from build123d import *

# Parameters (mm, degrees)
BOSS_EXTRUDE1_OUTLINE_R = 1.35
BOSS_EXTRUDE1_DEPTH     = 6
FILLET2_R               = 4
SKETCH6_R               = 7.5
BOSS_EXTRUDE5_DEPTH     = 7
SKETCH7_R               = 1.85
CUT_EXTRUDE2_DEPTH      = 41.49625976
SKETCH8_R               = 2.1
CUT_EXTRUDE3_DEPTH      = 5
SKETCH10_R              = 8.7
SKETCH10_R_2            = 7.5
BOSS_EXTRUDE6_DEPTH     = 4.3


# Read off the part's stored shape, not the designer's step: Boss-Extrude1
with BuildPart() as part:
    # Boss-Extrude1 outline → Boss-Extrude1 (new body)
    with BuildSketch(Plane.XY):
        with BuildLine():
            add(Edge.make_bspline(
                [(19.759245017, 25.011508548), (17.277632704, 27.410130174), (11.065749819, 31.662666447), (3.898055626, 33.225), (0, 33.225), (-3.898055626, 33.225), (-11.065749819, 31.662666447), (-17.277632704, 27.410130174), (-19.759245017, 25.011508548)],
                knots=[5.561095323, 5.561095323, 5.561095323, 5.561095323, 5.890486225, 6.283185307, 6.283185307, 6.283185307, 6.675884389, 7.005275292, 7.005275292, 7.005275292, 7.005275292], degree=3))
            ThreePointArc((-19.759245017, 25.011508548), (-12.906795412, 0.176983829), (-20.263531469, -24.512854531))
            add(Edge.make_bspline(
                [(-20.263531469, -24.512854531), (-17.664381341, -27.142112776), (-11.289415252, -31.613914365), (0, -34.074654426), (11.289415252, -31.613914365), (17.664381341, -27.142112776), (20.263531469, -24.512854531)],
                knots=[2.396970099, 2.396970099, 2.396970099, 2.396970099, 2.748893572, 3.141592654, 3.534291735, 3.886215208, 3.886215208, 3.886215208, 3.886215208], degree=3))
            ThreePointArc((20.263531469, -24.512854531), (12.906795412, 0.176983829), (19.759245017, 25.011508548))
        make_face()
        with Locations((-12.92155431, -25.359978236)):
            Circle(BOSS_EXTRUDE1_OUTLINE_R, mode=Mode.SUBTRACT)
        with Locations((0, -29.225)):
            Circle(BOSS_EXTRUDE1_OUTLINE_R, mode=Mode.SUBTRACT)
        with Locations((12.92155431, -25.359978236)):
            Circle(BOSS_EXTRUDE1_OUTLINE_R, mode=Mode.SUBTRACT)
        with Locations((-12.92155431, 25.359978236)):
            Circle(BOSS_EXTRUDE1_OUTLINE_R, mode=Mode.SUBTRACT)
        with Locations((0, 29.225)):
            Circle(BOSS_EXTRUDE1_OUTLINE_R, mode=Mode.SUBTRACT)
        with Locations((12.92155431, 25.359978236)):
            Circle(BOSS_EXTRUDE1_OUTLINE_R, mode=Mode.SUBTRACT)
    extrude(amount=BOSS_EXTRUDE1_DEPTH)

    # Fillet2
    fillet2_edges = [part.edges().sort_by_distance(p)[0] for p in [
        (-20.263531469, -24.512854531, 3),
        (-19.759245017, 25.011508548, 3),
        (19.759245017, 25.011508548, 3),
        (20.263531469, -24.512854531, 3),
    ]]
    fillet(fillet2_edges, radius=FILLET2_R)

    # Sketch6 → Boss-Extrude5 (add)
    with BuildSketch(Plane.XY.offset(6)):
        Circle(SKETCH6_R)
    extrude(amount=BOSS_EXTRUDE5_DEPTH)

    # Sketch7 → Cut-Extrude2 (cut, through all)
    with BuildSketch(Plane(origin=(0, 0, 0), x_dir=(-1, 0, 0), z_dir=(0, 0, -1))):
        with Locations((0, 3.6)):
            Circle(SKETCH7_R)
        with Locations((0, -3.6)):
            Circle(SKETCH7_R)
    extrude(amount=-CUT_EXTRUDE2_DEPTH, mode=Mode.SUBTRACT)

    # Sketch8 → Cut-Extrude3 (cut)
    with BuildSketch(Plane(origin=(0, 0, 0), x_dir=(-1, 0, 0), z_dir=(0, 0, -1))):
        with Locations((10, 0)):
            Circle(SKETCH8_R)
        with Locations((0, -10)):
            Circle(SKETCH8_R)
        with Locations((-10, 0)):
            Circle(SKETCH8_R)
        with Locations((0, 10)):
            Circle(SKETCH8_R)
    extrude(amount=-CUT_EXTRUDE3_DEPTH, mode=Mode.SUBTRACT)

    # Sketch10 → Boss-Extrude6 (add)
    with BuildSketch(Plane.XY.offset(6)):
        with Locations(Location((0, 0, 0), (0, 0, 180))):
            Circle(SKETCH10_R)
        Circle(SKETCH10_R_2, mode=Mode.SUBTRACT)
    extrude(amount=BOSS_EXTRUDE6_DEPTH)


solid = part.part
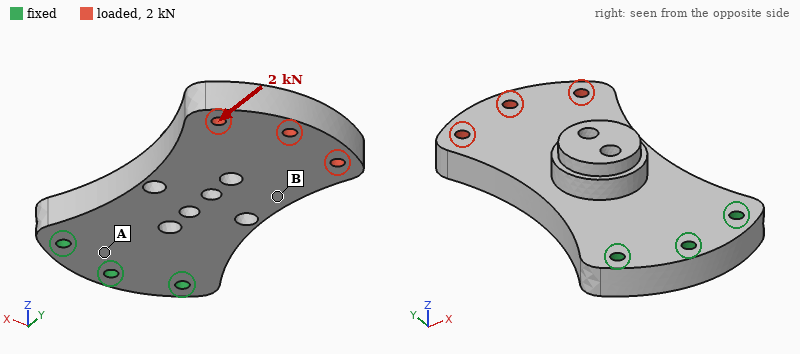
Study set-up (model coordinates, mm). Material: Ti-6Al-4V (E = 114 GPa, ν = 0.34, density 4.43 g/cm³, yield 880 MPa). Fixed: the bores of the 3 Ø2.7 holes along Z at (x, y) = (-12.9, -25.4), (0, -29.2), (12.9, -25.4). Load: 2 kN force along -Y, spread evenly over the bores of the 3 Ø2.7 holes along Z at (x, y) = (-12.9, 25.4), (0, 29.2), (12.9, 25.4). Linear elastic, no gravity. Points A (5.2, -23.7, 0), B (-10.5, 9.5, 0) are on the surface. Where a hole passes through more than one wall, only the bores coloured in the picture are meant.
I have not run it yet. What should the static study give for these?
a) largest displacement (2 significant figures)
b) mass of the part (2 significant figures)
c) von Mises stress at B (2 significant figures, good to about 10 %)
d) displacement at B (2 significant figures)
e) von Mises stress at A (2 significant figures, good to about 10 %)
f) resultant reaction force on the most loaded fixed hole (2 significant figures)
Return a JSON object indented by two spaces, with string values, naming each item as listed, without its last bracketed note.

{
  "largest displacement": "12 µm",
  "mass of the part": "55 g",
  "von Mises stress at B": "13 MPa",
  "displacement at B": "5.9 µm",
  "von Mises stress at A": "5.7 MPa",
  "resultant reaction force on the most loaded fixed hole": "720 N"
}
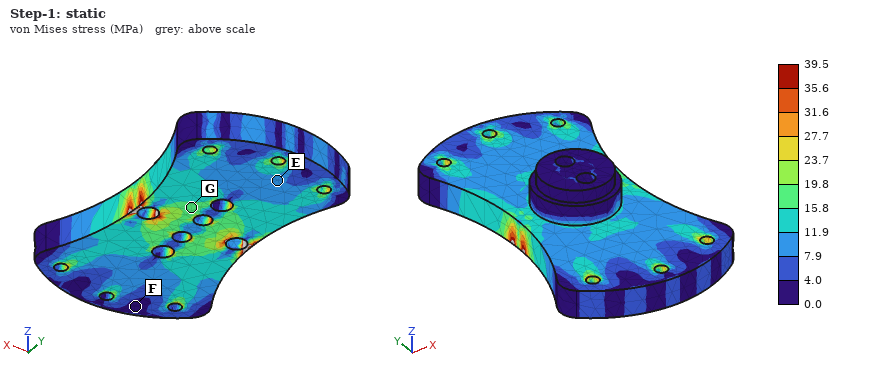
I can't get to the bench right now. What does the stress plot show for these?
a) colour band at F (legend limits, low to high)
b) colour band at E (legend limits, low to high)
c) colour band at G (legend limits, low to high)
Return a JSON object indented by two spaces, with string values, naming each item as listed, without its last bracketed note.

{
  "colour band at F": "0.0 to 4.0 MPa",
  "colour band at E": "7.9 to 11.9 MPa",
  "colour band at G": "15.8 to 19.8 MPa"
}
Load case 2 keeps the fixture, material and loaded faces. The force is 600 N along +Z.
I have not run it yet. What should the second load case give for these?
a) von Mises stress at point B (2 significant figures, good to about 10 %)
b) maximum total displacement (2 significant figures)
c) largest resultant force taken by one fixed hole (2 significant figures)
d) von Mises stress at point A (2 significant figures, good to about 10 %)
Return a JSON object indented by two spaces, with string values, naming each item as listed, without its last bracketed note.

{
  "von Mises stress at point B": "57 MPa",
  "maximum total displacement": "0.54 mm",
  "largest resultant force taken by one fixed hole": "470 N",
  "von Mises stress at point A": "94 MPa"
}
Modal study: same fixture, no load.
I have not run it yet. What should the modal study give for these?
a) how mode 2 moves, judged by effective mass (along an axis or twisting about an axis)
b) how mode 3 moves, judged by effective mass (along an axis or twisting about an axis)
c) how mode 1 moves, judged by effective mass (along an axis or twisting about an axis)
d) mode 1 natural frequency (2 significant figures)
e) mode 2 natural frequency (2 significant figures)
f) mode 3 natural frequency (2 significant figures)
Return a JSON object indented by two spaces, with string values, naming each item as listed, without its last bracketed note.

{
  "how mode 2 moves, judged by effective mass": "along X",
  "how mode 3 moves, judged by effective mass": "along X",
  "how mode 1 moves, judged by effective mass": "along Z",
  "mode 1 natural frequency": "1400 Hz",
  "mode 2 natural frequency": "5600 Hz",
  "mode 3 natural frequency": "6000 Hz"
}
